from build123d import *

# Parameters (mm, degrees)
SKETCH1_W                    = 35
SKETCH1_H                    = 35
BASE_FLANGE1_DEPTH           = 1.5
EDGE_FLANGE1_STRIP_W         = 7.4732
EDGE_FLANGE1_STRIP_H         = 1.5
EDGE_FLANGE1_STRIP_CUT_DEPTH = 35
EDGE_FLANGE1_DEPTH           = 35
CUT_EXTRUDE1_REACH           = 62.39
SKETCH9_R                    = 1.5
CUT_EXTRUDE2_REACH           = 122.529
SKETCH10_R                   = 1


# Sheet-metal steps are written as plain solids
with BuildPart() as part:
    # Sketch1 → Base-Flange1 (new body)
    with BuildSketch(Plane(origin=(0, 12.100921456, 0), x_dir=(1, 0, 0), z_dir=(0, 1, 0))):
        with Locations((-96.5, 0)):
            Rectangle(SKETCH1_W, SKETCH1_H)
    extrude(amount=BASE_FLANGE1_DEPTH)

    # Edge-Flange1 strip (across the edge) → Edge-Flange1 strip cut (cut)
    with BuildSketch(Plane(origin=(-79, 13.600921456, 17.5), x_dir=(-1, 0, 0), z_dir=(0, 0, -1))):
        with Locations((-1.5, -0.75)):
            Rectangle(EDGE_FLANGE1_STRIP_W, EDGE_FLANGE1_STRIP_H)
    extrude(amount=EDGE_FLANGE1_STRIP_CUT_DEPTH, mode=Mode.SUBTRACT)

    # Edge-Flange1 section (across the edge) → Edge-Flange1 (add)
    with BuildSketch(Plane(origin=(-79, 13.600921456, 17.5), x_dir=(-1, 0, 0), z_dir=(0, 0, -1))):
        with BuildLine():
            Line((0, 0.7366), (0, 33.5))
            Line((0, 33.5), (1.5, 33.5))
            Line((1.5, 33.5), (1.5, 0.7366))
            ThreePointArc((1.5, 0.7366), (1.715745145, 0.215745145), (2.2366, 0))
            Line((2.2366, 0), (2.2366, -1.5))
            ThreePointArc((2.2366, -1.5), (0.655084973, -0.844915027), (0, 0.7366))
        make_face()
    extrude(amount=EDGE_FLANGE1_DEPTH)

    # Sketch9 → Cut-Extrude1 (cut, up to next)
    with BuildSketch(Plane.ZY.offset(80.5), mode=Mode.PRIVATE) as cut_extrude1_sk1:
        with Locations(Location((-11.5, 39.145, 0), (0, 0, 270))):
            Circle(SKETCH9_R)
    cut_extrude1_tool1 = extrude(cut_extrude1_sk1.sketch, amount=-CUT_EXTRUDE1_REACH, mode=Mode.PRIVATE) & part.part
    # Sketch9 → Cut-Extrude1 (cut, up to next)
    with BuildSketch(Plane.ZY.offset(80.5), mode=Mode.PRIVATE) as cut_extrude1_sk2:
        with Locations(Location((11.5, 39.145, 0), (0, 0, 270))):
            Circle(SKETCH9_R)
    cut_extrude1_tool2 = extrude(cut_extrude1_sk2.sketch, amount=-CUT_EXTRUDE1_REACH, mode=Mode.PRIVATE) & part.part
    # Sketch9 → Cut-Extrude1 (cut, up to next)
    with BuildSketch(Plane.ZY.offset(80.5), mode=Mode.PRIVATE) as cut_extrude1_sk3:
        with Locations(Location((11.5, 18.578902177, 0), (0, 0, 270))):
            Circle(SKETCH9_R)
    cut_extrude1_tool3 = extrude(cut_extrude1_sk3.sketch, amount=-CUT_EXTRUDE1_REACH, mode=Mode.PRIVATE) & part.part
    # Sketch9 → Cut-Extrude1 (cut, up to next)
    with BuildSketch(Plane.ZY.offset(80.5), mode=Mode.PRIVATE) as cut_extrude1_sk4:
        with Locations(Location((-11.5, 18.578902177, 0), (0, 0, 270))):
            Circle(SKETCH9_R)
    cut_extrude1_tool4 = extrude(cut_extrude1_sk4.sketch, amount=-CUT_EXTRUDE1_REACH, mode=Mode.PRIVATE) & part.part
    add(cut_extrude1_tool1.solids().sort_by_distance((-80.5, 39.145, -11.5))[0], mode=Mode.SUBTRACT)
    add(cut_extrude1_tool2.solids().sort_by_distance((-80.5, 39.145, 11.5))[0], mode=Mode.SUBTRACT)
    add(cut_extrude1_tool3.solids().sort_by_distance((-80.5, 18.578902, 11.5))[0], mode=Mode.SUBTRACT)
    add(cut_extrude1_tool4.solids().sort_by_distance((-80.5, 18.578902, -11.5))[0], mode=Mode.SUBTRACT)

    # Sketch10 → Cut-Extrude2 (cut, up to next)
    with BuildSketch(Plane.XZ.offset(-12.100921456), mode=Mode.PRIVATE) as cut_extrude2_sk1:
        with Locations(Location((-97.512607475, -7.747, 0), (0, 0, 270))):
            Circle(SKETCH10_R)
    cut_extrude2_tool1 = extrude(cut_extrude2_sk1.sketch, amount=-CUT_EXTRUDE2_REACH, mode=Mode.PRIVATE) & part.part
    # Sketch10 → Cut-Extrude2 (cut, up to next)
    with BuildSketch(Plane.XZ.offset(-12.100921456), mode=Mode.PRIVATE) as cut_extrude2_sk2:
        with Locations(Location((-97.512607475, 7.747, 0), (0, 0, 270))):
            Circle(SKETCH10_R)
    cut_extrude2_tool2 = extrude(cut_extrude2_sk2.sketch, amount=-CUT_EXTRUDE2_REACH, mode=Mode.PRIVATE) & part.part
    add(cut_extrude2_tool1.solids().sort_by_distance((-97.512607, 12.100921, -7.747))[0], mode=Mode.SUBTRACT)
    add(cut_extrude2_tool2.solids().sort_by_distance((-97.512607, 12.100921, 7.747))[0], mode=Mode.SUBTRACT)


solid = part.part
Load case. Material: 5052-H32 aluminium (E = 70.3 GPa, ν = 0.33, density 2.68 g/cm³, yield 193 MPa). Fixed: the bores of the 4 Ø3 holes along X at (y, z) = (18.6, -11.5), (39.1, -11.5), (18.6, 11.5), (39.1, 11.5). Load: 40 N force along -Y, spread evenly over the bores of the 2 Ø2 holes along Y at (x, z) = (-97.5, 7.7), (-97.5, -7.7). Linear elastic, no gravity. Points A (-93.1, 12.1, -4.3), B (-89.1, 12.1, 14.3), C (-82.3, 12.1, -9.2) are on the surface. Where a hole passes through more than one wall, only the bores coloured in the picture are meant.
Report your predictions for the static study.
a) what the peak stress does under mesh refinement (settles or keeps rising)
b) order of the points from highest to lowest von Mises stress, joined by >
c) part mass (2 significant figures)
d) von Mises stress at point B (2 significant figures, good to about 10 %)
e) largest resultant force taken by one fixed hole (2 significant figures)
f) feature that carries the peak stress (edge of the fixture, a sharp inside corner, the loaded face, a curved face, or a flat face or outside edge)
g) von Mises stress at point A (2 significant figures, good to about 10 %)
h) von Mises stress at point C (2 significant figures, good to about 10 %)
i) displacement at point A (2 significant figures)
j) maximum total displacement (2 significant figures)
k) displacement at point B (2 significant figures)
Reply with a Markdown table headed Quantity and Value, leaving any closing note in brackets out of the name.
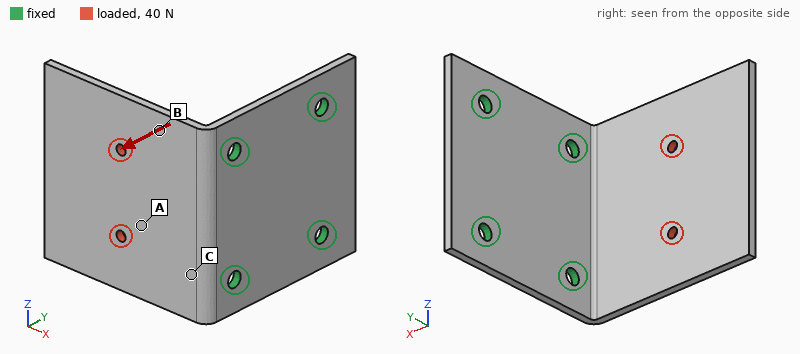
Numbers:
| Quantity | Value |
|---|---|
| what the peak stress does under mesh refinement | keeps rising |
| order of the points from highest to lowest von Mises stress, joined by > | C > B > A |
| part mass | 9.4 g |
| von Mises stress at point B | 25 MPa |
| largest resultant force taken by one fixed hole | 16 N |
| feature that carries the peak stress | edge of the fixture |
| von Mises stress at point A | 12 MPa |
| von Mises stress at point C | 42 MPa |
| displacement at point A | 0.13 mm |
| maximum total displacement | 0.41 mm |
| displacement at point B | 0.080 mm |
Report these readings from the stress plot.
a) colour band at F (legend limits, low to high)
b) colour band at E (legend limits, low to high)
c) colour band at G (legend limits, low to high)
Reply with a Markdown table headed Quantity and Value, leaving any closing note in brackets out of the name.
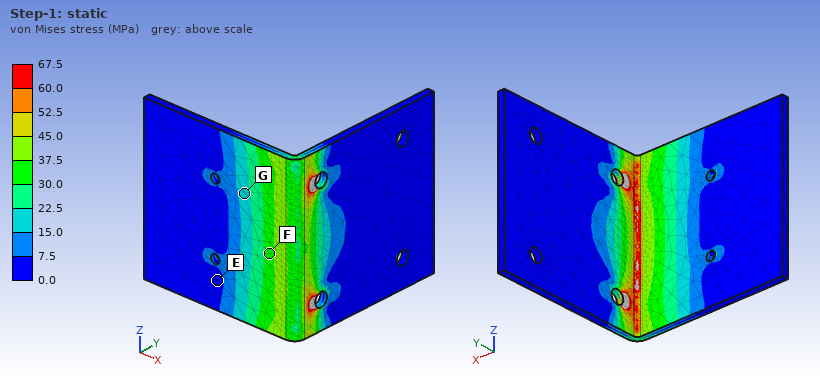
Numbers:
| Quantity | Value |
|---|---|
| colour band at F | 30.0 to 37.5 MPa |
| colour band at E | 0.0 to 7.5 MPa |
| colour band at G | 15.0 to 22.5 MPa |
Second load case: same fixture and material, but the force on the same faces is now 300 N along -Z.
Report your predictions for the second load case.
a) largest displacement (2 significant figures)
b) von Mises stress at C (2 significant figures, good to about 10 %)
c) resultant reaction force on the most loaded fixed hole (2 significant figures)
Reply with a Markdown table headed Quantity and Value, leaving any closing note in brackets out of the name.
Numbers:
| Quantity | Value |
|---|---|
| largest displacement | 0.14 mm |
| von Mises stress at C | 25 MPa |
| resultant reaction force on the most loaded fixed hole | 270 N |
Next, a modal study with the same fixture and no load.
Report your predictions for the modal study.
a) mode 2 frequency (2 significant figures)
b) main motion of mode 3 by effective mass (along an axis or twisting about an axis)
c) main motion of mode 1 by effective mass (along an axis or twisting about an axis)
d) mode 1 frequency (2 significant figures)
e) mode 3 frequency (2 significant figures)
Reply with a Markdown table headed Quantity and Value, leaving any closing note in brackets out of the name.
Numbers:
| Quantity | Value |
|---|---|
| mode 2 frequency | 2300 Hz |
| main motion of mode 3 by effective mass | along Z |
| main motion of mode 1 by effective mass | along Y |
| mode 1 frequency | 870 Hz |
| mode 3 frequency | 4800 Hz |
